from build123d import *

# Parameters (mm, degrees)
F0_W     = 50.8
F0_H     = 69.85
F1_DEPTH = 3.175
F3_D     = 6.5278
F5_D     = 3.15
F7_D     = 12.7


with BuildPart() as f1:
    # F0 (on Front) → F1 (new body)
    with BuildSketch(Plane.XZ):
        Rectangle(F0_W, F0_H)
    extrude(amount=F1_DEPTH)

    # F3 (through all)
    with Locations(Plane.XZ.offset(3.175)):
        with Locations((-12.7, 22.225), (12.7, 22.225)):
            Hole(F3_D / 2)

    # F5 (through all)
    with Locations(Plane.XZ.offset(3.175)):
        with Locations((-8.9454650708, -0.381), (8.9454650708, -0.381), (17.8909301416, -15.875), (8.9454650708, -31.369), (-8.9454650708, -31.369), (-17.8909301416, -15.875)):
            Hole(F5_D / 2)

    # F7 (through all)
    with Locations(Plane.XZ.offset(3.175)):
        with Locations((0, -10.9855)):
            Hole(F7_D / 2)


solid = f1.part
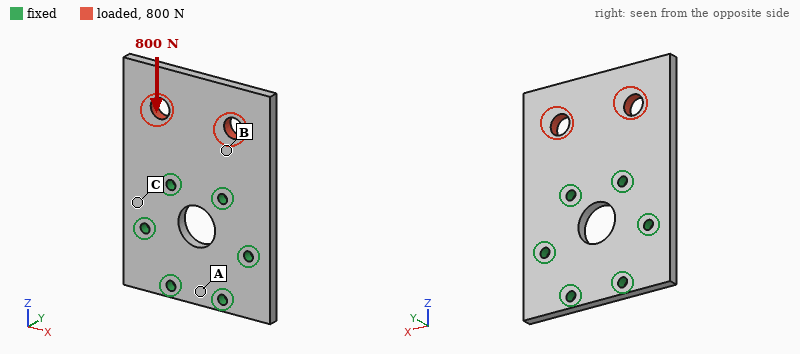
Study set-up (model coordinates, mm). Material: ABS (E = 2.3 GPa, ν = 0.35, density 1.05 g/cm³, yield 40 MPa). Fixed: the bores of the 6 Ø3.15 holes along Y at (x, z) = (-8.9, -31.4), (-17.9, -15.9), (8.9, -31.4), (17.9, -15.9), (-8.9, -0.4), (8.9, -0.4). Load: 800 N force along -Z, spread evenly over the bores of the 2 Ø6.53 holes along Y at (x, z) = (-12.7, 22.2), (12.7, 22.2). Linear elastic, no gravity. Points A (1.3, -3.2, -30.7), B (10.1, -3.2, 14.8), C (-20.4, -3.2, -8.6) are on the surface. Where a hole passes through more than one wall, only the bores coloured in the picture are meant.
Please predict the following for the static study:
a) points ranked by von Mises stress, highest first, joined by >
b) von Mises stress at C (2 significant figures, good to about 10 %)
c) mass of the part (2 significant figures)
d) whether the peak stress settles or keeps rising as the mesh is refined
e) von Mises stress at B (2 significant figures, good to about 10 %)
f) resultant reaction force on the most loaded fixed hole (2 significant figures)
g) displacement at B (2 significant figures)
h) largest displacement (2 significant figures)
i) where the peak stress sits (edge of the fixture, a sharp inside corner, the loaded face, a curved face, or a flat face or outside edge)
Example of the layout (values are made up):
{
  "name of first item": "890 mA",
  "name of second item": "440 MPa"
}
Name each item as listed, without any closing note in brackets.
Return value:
{
  "points ranked by von Mises stress, highest first, joined by >": "B > C > A",
  "von Mises stress at C": "3.4 MPa",
  "mass of the part": "11 g",
  "whether the peak stress settles or keeps rising as the mesh is refined": "keeps rising",
  "von Mises stress at B": "6.7 MPa",
  "resultant reaction force on the most loaded fixed hole": "280 N",
  "displacement at B": "48 µm",
  "largest displacement": "89 µm",
  "where the peak stress sits": "edge of the fixture"
}
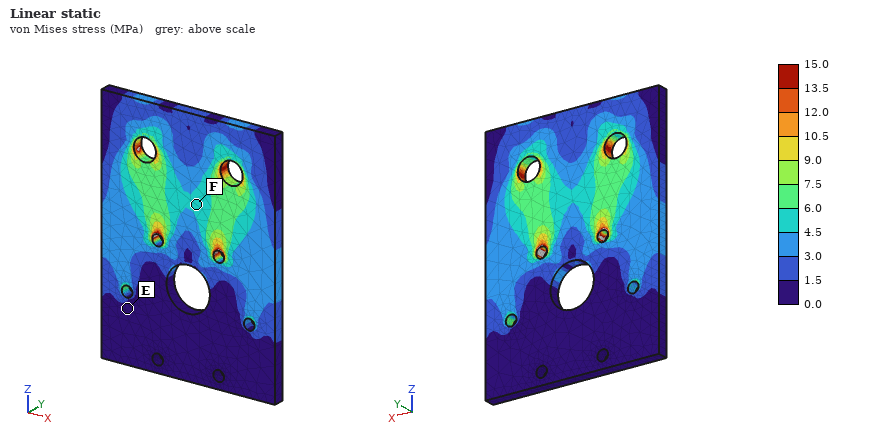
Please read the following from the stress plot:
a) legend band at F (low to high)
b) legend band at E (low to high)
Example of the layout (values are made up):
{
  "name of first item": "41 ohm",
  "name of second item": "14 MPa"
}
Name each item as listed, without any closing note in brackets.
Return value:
{
  "legend band at F": "4.5 to 6.0 MPa",
  "legend band at E": "0.0 to 1.5 MPa"
}
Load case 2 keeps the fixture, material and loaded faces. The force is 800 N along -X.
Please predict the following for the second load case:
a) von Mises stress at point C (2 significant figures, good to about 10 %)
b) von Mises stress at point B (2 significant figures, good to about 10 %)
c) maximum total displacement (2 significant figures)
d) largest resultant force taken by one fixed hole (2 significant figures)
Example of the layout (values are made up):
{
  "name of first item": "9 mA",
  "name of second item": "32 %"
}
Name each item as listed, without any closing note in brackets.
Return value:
{
  "von Mises stress at point C": "9.5 MPa",
  "von Mises stress at point B": "12 MPa",
  "maximum total displacement": "0.39 mm",
  "largest resultant force taken by one fixed hole": "540 N"
}
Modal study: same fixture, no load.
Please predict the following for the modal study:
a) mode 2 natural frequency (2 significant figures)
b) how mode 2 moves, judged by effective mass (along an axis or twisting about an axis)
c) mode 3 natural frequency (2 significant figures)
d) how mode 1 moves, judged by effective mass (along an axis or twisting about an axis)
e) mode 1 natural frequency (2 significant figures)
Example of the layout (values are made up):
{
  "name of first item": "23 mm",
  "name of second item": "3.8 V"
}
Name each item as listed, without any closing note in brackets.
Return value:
{
  "mode 2 natural frequency": "970 Hz",
  "how mode 2 moves, judged by effective mass": "twisting about Z",
  "mode 3 natural frequency": "2200 Hz",
  "how mode 1 moves, judged by effective mass": "along Y",
  "mode 1 natural frequency": "600 Hz"
}
